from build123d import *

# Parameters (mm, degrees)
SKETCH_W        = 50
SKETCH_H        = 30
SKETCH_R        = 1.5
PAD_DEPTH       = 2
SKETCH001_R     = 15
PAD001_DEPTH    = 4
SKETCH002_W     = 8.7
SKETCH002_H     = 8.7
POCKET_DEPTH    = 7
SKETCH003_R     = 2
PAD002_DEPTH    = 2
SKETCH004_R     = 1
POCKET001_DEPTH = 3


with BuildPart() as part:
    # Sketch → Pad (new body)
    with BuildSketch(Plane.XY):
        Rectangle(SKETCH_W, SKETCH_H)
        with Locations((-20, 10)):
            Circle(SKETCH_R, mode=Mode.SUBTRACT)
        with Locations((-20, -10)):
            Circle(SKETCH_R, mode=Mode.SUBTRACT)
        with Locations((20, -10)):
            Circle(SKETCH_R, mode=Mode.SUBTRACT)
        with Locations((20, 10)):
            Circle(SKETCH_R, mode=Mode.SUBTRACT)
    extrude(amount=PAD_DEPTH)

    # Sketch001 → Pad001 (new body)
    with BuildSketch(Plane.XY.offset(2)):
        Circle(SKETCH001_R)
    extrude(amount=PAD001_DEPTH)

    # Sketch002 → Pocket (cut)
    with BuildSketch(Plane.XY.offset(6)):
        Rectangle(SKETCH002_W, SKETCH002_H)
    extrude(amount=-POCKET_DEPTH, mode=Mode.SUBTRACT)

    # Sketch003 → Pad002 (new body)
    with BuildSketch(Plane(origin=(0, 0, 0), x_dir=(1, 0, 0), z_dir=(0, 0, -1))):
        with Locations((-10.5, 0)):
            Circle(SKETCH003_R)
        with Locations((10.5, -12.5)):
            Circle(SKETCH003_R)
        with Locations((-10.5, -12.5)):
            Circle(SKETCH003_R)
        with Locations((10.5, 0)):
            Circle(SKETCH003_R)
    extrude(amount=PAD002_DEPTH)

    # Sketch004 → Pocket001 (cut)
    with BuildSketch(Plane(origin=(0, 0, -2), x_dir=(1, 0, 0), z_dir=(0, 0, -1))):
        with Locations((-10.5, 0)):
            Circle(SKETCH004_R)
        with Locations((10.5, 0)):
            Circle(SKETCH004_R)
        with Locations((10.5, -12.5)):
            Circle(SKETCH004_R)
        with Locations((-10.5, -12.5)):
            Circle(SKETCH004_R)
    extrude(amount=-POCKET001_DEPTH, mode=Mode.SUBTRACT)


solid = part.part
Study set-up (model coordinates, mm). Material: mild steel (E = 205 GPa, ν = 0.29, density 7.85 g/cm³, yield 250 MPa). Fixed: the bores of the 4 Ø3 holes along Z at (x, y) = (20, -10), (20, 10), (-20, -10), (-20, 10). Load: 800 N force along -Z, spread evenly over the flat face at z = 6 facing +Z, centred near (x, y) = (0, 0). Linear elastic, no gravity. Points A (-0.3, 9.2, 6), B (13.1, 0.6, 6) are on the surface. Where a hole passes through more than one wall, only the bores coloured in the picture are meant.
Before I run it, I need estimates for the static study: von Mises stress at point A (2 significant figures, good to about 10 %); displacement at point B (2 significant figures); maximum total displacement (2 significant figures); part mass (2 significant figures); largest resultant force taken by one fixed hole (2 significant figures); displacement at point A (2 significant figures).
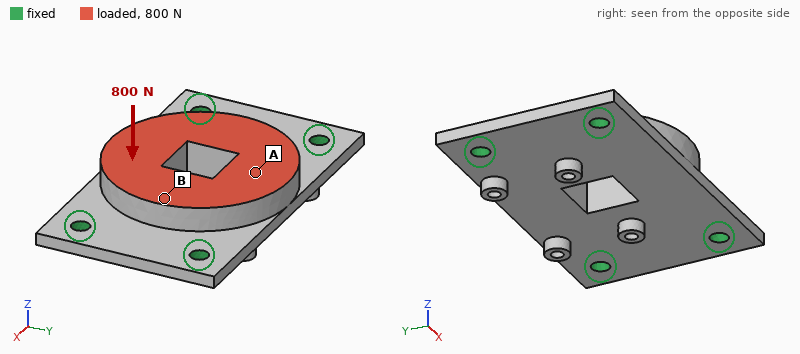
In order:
25 MPa
6.8 µm
10 µm
42 g
300 N
9.7 µm
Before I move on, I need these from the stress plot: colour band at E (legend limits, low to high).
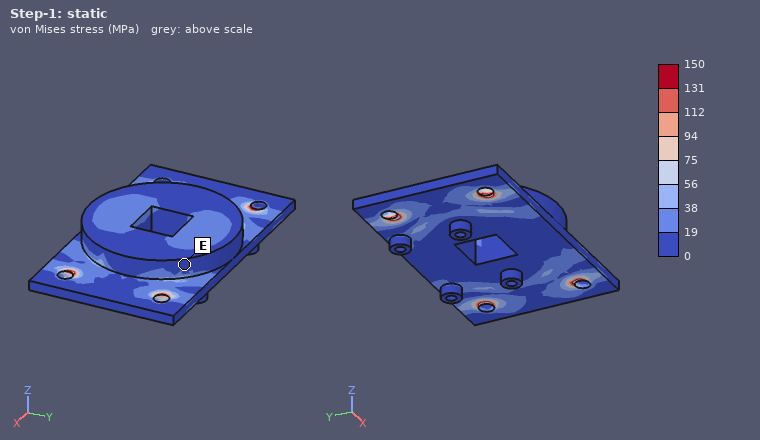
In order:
0 to 19 MPa
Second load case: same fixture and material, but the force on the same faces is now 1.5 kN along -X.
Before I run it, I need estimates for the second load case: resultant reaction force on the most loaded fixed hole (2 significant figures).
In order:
400 N
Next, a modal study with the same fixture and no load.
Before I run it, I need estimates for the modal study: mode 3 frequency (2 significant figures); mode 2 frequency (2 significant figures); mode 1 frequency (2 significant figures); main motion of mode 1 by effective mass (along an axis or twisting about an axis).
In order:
18 kHz
9700 Hz
8400 Hz
along Z
